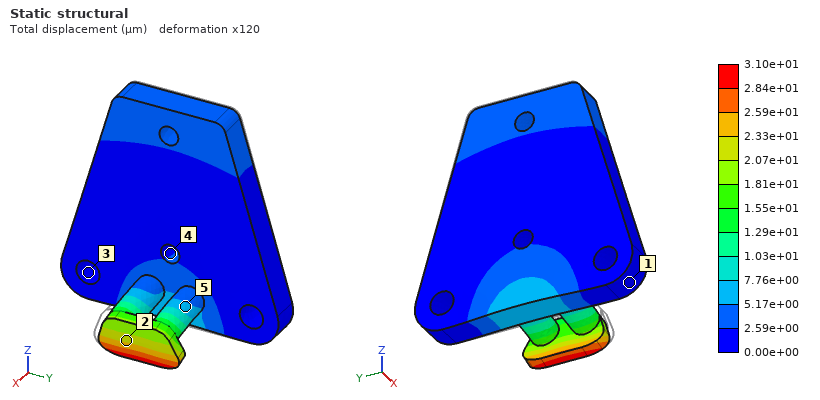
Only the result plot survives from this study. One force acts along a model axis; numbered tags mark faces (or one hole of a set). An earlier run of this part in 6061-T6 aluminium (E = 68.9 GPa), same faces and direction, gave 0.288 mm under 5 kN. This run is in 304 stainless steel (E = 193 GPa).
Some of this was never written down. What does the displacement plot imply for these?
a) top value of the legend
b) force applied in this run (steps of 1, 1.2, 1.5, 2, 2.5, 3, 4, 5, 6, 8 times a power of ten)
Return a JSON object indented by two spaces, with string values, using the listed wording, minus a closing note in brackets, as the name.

{
  "top value of the legend": "3.10e+01 µm",
  "force applied in this run": "1.5 kN"
}
